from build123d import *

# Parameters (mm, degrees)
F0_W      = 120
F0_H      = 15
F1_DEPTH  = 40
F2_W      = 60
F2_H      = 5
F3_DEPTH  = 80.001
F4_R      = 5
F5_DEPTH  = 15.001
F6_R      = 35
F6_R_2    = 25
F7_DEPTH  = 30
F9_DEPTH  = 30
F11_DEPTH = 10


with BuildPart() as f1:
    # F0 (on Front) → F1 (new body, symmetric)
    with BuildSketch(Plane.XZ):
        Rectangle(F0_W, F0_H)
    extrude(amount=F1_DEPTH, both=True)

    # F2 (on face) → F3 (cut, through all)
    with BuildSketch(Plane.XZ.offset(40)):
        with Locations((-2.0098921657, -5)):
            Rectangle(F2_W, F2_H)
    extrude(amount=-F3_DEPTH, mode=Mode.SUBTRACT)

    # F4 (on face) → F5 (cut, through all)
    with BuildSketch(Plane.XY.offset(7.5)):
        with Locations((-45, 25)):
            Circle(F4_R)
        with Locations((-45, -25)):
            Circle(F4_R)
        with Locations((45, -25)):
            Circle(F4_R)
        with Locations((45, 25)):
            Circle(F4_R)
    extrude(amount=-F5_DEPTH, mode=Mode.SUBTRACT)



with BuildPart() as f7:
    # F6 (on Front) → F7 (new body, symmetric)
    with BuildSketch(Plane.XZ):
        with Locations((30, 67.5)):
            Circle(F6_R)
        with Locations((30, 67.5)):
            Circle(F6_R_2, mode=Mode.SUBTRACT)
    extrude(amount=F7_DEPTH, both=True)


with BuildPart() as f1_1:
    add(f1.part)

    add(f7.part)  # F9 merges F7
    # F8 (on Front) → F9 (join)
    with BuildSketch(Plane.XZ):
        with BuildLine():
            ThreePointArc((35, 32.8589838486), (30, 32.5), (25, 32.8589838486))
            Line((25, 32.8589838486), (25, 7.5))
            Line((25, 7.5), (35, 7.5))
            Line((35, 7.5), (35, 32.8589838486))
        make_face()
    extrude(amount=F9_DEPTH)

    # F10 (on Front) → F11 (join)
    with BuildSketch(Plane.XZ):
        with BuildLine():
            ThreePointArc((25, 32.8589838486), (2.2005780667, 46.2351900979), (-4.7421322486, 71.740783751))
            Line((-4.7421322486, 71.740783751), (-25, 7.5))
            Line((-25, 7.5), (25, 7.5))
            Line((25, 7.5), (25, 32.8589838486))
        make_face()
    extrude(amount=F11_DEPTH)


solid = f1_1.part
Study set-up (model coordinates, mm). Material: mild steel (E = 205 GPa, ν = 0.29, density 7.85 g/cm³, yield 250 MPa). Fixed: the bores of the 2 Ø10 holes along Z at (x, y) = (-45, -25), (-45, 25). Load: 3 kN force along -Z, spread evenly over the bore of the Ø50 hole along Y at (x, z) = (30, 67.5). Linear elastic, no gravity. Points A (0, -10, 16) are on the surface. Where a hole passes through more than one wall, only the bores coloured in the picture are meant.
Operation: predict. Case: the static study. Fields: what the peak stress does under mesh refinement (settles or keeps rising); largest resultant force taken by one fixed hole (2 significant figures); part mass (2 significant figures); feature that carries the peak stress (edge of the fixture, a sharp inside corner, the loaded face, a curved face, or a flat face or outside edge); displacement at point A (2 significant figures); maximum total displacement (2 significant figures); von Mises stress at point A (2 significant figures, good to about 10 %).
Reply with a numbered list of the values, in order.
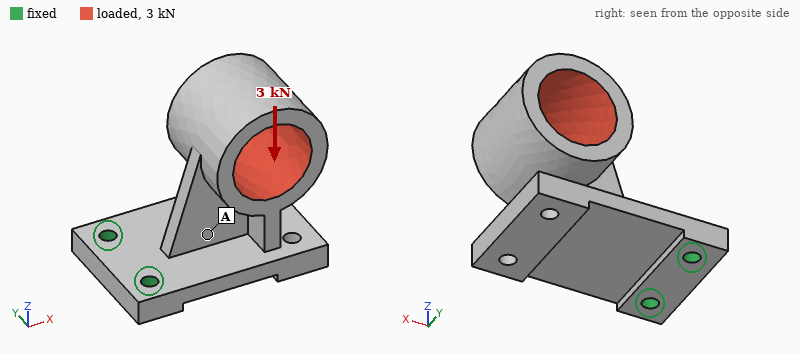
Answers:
1. keeps rising
2. 1.6 kN
3. 2.0 kg
4. edge of the fixture
5. 0.098 mm
6. 0.42 mm
7. 17 MPa
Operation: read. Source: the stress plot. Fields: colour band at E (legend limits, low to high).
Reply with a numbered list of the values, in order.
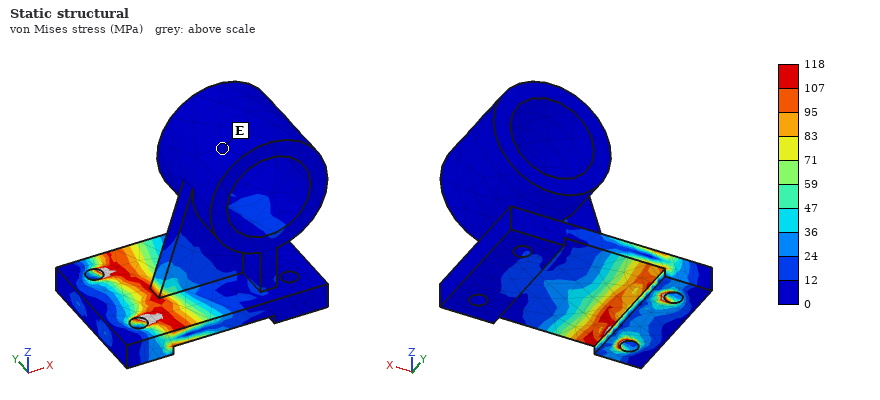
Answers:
1. 0 to 12 MPa
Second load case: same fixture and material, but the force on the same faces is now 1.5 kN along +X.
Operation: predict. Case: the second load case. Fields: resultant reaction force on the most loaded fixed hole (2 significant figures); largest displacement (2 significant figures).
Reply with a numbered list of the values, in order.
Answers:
1. 830 N
2. 0.24 mm
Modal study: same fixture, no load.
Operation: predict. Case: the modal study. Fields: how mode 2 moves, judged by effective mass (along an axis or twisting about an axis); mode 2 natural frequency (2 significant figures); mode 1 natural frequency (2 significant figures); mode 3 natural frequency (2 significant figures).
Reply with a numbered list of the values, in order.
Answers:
1. along Y
2. 530 Hz
3. 370 Hz
4. 1800 Hz
